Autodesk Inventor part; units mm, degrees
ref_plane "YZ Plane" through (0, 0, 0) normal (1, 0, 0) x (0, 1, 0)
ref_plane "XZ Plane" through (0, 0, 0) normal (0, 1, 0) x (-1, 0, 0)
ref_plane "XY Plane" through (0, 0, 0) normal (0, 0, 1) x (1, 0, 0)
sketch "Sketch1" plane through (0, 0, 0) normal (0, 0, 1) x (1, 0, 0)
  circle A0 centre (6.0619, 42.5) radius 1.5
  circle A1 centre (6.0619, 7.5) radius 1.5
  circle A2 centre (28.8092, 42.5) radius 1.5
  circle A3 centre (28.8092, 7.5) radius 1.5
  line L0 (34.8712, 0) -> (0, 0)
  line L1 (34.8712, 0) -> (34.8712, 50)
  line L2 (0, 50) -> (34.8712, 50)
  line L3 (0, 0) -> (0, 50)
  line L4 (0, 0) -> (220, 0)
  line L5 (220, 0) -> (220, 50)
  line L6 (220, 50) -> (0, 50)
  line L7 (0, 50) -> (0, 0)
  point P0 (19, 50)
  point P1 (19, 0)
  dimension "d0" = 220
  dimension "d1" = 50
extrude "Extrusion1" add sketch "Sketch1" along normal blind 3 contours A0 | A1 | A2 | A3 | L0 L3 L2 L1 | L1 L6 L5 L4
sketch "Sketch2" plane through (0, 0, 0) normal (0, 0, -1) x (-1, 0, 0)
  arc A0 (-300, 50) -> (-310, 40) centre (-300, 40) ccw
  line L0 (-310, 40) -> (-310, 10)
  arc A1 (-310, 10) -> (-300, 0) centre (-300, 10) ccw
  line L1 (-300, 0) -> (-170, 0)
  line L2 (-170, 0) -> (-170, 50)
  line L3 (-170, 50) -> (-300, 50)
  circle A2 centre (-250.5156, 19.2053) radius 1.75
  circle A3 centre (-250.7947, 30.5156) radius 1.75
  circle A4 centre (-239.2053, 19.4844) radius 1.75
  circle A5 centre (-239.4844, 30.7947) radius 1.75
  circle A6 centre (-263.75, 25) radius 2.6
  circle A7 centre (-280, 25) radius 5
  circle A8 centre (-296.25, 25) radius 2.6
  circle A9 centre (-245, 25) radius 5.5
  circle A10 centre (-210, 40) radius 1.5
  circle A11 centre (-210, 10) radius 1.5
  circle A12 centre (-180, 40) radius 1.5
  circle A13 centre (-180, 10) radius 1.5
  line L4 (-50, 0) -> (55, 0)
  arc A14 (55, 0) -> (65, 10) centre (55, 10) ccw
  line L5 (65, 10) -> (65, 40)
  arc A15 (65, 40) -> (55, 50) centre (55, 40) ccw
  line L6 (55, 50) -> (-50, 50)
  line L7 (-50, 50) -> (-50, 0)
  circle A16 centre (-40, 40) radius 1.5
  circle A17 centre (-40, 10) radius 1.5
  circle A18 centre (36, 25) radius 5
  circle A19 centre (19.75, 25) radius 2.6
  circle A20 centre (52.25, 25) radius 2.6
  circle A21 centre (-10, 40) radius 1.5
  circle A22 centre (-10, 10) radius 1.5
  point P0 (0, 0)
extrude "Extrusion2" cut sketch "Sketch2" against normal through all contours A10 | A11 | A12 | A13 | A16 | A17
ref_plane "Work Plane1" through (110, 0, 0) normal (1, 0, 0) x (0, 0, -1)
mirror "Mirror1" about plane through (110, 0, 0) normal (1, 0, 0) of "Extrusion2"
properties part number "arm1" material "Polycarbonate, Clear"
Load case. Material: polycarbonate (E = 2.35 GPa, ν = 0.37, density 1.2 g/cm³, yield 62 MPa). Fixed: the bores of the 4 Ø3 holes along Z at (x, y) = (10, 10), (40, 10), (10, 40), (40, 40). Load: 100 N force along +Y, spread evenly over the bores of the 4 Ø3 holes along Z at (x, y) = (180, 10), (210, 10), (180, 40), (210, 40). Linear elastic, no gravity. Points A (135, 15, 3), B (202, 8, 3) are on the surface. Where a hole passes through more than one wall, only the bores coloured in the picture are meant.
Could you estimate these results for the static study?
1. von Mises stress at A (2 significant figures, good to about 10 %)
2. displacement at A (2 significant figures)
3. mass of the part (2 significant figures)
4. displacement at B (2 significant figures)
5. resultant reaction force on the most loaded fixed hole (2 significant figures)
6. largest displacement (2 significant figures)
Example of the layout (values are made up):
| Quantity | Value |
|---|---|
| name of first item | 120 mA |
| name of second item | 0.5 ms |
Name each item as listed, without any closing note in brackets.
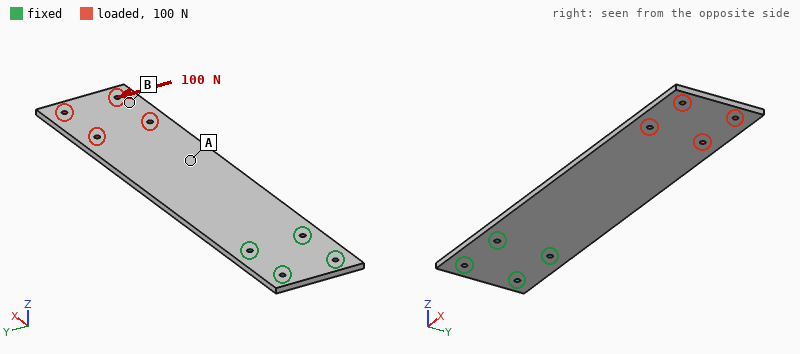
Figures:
| Quantity | Value |
|---|---|
| von Mises stress at A | 2.4 MPa |
| displacement at A | 0.98 mm |
| mass of the part | 39 g |
| displacement at B | 2.2 mm |
| resultant reaction force on the most loaded fixed hole | 380 N |
| largest displacement | 2.5 mm |
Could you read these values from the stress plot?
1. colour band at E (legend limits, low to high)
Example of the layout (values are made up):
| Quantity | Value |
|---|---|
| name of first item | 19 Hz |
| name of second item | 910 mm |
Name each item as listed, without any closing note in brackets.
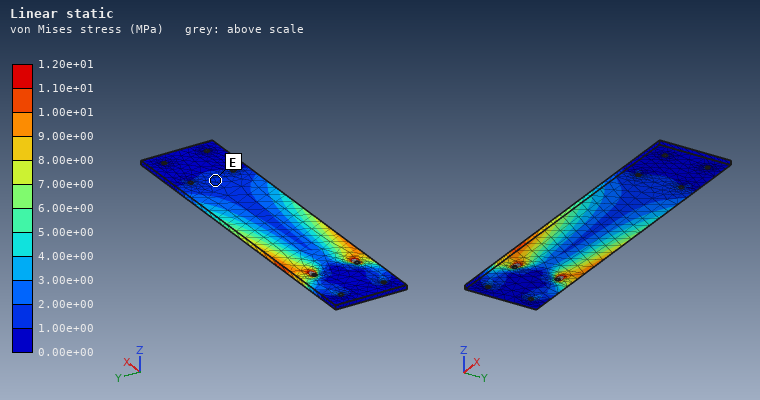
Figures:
| Quantity | Value |
|---|---|
| colour band at E | 1.00e+00 to 2.00e+00 MPa |
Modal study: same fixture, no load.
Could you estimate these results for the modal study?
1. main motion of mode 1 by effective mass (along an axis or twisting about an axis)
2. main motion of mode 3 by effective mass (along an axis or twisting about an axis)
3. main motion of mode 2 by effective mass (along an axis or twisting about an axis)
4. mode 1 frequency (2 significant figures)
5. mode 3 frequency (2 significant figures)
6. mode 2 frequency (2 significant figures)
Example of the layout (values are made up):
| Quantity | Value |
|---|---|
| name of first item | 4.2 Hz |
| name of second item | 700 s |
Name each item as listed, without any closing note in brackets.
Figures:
| Quantity | Value |
|---|---|
| main motion of mode 1 by effective mass | along Z |
| main motion of mode 3 by effective mass | twisting about X |
| main motion of mode 2 by effective mass | along Z |
| mode 1 frequency | 21 Hz |
| mode 3 frequency | 150 Hz |
| mode 2 frequency | 130 Hz |
